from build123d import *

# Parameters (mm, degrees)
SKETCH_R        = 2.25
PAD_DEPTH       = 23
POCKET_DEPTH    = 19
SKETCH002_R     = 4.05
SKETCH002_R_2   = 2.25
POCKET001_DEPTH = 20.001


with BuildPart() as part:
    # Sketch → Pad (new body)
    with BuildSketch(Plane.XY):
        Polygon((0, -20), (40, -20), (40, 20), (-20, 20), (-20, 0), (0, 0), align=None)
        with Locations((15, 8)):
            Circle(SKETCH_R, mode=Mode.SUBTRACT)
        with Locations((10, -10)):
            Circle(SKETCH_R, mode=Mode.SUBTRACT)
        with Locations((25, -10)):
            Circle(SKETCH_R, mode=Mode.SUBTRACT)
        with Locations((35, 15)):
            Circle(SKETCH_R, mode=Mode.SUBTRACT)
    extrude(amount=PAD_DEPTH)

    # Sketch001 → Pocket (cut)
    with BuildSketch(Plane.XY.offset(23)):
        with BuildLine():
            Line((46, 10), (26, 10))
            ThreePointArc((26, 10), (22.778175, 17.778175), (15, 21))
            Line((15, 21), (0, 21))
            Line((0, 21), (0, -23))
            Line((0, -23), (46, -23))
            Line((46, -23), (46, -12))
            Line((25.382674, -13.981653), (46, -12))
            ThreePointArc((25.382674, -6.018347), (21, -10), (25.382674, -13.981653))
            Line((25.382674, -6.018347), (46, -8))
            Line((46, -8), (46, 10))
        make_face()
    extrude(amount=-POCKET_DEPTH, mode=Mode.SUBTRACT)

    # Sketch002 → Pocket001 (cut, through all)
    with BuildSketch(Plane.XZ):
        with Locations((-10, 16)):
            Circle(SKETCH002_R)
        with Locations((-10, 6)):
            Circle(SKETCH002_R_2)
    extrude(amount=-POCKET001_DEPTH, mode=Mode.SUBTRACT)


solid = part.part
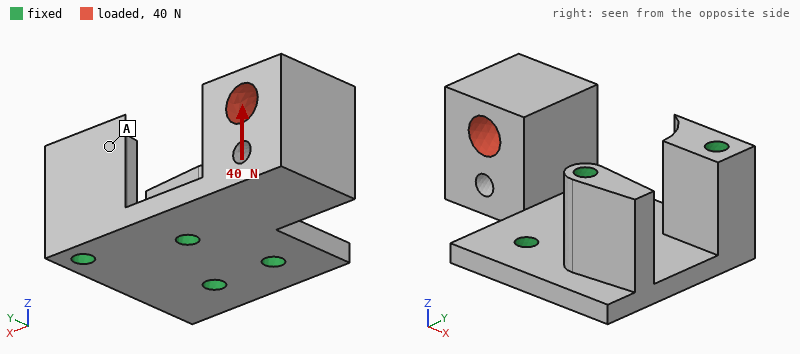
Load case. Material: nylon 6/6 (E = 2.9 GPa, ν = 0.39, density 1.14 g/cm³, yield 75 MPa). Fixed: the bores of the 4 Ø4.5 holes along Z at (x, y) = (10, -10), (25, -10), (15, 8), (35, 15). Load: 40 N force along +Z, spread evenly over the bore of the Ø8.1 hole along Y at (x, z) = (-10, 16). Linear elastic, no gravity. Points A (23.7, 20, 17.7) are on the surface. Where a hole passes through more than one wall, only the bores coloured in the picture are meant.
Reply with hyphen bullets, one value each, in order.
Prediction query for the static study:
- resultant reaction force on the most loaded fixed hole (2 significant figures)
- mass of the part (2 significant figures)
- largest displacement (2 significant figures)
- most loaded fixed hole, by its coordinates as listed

- 47 N
- 21 g
- 0.87 mm
- (15, 8)
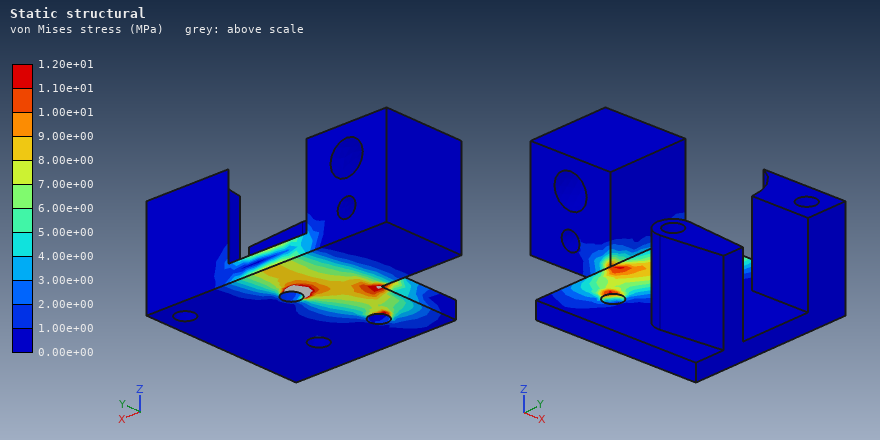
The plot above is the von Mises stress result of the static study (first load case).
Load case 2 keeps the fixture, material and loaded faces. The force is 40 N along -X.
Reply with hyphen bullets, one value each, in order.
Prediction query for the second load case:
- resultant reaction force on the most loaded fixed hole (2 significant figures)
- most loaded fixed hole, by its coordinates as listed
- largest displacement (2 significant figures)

- 33 N
- (15, 8)
- 0.73 mm
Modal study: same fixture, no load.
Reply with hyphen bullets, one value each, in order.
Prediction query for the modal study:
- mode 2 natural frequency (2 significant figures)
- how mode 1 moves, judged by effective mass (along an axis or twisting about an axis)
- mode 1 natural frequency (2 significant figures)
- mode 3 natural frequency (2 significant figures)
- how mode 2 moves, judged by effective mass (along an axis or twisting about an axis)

- 1000 Hz
- along Z
- 410 Hz
- 2500 Hz
- along Y
